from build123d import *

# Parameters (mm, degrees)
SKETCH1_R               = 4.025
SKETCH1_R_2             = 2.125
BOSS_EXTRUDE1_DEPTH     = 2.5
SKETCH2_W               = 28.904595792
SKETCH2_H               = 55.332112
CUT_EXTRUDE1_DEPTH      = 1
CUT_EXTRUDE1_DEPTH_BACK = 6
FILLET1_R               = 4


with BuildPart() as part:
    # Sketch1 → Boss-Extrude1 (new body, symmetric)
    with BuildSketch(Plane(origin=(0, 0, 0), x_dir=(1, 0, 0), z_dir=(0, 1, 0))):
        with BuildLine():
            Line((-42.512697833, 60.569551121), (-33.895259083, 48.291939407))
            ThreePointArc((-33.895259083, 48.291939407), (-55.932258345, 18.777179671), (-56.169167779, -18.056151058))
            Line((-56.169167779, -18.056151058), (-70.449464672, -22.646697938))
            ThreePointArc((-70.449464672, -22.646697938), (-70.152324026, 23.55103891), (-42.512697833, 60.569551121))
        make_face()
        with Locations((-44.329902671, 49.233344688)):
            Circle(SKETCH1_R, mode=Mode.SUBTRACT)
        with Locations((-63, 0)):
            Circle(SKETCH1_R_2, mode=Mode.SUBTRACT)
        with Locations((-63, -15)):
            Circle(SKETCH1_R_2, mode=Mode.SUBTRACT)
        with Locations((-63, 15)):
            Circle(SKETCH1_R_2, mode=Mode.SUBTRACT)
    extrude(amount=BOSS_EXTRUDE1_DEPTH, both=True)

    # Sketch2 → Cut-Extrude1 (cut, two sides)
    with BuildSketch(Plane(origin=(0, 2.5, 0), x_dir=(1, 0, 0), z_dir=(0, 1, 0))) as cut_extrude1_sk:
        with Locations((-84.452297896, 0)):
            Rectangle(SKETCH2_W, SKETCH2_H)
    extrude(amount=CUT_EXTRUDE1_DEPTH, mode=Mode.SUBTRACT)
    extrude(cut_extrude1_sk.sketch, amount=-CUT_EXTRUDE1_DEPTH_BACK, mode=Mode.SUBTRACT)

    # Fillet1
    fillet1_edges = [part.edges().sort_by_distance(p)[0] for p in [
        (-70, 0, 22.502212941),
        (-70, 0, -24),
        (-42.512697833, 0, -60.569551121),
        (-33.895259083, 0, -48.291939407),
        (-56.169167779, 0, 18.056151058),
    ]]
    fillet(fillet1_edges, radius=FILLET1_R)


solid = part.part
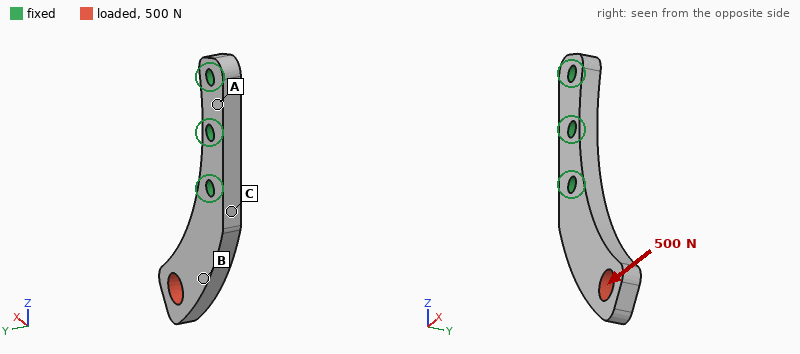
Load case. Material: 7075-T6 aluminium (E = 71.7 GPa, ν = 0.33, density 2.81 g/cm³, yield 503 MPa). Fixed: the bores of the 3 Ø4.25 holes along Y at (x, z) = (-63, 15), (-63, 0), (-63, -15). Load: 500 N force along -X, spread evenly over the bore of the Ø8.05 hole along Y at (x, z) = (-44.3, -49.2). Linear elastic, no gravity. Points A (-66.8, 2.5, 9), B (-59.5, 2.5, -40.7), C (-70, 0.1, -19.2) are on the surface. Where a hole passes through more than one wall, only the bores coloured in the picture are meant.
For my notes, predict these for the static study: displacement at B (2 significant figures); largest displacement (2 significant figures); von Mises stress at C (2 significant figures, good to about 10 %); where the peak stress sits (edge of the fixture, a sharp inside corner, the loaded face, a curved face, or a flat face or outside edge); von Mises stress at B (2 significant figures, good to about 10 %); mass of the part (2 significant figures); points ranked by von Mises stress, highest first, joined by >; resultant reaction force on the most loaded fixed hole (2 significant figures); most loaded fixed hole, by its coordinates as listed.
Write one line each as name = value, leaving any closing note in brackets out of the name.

displacement at B = 0.085 mm
largest displacement = 0.19 mm
von Mises stress at C = 90 MPa
where the peak stress sits = edge of the fixture
von Mises stress at B = 27 MPa
mass of the part = 14 g
points ranked by von Mises stress, highest first, joined by > = C > B > A
resultant reaction force on the most loaded fixed hole = 1.0 kN
most loaded fixed hole, by its coordinates as listed = (-63, -15)
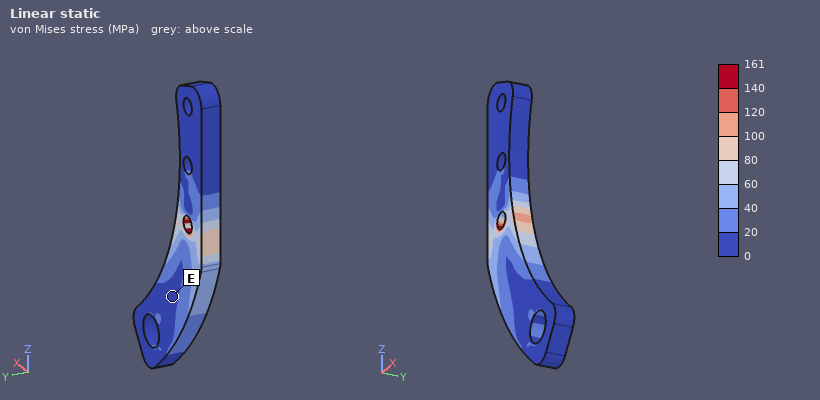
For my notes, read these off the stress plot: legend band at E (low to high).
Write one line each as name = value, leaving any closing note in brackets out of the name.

legend band at E = 0 to 20 MPa
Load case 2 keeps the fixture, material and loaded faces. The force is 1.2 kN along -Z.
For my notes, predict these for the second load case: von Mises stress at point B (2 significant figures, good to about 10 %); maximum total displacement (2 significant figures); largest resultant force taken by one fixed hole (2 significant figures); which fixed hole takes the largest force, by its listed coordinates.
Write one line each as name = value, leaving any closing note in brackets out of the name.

von Mises stress at point B = 37 MPa
maximum total displacement = 0.30 mm
largest resultant force taken by one fixed hole = 1.5 kN
which fixed hole takes the largest force, by its listed coordinates = (-63, -15)
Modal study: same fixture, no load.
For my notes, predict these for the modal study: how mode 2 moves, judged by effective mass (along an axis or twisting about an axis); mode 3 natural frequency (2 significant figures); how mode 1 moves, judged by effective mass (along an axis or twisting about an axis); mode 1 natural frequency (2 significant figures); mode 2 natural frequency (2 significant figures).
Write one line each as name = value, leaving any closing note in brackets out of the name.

how mode 2 moves, judged by effective mass = along X
mode 3 natural frequency = 8500 Hz
how mode 1 moves, judged by effective mass = along Y
mode 1 natural frequency = 2000 Hz
mode 2 natural frequency = 4400 Hz
